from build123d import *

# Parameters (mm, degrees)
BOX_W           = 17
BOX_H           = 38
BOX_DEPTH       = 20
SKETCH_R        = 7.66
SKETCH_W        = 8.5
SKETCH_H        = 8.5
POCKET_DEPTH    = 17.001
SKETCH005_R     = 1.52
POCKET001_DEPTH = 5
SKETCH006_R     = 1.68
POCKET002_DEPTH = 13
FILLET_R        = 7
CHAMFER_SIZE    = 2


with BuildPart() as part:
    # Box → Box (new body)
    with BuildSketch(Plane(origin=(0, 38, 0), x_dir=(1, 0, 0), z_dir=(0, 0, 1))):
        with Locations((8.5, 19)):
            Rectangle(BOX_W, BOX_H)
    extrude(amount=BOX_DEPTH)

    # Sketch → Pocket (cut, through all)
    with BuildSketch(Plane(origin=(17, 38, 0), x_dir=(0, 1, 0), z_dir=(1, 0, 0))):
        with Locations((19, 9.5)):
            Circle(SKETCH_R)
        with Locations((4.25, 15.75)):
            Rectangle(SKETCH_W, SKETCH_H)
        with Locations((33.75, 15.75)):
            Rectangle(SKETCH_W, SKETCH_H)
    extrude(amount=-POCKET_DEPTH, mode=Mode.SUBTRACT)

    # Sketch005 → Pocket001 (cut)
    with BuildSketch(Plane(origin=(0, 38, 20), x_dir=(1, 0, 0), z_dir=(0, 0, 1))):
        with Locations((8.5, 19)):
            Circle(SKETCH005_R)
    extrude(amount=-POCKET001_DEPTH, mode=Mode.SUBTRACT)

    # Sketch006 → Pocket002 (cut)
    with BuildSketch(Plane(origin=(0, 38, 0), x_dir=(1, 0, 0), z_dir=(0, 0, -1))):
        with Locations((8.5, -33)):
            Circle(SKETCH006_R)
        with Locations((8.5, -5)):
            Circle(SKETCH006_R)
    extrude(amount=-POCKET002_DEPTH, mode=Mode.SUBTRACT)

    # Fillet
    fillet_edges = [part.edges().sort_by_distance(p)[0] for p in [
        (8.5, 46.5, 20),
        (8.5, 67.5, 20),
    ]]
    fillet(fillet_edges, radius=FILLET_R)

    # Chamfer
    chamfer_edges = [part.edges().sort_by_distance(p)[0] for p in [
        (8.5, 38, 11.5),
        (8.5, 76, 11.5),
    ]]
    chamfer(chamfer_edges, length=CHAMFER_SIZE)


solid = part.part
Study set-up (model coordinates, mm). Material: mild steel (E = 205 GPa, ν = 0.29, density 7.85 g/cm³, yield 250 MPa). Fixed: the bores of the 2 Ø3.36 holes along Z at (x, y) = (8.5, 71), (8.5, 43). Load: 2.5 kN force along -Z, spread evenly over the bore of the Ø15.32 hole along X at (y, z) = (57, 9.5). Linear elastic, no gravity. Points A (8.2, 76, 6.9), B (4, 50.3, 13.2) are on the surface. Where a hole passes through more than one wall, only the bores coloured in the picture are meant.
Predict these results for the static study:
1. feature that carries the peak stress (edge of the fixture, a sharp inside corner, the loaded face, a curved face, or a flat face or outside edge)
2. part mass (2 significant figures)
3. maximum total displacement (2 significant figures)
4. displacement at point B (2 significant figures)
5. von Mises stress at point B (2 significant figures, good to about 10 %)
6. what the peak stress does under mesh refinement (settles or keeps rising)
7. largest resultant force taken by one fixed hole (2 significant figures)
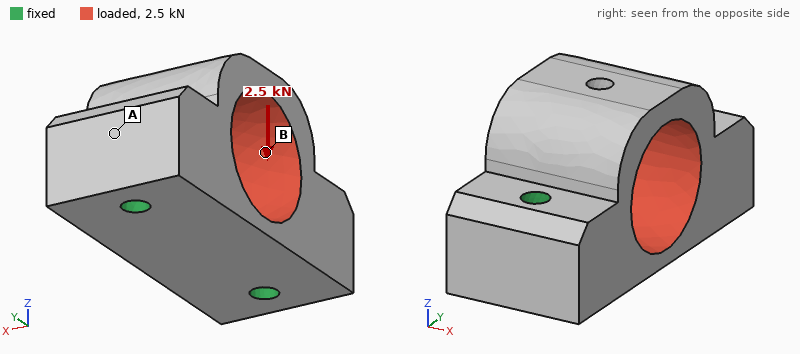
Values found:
edge of the fixture
52 g
2.1 µm
1.0 µm
14 MPa
keeps rising
1.3 kN
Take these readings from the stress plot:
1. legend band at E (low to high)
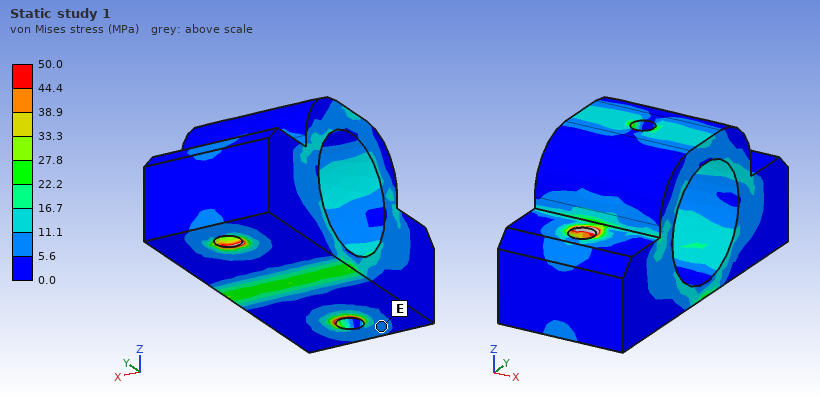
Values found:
5.6 to 11.1 MPa
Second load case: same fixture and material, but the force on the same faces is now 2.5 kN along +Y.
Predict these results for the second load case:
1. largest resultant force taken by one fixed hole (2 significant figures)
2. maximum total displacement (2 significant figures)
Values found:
1.3 kN
2.5 µm
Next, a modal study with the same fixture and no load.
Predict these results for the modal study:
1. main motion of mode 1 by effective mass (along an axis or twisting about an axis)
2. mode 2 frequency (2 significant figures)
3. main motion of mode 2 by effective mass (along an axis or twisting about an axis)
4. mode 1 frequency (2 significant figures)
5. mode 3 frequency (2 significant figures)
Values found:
along X
31 kHz
along Y
25 kHz
38 kHz
